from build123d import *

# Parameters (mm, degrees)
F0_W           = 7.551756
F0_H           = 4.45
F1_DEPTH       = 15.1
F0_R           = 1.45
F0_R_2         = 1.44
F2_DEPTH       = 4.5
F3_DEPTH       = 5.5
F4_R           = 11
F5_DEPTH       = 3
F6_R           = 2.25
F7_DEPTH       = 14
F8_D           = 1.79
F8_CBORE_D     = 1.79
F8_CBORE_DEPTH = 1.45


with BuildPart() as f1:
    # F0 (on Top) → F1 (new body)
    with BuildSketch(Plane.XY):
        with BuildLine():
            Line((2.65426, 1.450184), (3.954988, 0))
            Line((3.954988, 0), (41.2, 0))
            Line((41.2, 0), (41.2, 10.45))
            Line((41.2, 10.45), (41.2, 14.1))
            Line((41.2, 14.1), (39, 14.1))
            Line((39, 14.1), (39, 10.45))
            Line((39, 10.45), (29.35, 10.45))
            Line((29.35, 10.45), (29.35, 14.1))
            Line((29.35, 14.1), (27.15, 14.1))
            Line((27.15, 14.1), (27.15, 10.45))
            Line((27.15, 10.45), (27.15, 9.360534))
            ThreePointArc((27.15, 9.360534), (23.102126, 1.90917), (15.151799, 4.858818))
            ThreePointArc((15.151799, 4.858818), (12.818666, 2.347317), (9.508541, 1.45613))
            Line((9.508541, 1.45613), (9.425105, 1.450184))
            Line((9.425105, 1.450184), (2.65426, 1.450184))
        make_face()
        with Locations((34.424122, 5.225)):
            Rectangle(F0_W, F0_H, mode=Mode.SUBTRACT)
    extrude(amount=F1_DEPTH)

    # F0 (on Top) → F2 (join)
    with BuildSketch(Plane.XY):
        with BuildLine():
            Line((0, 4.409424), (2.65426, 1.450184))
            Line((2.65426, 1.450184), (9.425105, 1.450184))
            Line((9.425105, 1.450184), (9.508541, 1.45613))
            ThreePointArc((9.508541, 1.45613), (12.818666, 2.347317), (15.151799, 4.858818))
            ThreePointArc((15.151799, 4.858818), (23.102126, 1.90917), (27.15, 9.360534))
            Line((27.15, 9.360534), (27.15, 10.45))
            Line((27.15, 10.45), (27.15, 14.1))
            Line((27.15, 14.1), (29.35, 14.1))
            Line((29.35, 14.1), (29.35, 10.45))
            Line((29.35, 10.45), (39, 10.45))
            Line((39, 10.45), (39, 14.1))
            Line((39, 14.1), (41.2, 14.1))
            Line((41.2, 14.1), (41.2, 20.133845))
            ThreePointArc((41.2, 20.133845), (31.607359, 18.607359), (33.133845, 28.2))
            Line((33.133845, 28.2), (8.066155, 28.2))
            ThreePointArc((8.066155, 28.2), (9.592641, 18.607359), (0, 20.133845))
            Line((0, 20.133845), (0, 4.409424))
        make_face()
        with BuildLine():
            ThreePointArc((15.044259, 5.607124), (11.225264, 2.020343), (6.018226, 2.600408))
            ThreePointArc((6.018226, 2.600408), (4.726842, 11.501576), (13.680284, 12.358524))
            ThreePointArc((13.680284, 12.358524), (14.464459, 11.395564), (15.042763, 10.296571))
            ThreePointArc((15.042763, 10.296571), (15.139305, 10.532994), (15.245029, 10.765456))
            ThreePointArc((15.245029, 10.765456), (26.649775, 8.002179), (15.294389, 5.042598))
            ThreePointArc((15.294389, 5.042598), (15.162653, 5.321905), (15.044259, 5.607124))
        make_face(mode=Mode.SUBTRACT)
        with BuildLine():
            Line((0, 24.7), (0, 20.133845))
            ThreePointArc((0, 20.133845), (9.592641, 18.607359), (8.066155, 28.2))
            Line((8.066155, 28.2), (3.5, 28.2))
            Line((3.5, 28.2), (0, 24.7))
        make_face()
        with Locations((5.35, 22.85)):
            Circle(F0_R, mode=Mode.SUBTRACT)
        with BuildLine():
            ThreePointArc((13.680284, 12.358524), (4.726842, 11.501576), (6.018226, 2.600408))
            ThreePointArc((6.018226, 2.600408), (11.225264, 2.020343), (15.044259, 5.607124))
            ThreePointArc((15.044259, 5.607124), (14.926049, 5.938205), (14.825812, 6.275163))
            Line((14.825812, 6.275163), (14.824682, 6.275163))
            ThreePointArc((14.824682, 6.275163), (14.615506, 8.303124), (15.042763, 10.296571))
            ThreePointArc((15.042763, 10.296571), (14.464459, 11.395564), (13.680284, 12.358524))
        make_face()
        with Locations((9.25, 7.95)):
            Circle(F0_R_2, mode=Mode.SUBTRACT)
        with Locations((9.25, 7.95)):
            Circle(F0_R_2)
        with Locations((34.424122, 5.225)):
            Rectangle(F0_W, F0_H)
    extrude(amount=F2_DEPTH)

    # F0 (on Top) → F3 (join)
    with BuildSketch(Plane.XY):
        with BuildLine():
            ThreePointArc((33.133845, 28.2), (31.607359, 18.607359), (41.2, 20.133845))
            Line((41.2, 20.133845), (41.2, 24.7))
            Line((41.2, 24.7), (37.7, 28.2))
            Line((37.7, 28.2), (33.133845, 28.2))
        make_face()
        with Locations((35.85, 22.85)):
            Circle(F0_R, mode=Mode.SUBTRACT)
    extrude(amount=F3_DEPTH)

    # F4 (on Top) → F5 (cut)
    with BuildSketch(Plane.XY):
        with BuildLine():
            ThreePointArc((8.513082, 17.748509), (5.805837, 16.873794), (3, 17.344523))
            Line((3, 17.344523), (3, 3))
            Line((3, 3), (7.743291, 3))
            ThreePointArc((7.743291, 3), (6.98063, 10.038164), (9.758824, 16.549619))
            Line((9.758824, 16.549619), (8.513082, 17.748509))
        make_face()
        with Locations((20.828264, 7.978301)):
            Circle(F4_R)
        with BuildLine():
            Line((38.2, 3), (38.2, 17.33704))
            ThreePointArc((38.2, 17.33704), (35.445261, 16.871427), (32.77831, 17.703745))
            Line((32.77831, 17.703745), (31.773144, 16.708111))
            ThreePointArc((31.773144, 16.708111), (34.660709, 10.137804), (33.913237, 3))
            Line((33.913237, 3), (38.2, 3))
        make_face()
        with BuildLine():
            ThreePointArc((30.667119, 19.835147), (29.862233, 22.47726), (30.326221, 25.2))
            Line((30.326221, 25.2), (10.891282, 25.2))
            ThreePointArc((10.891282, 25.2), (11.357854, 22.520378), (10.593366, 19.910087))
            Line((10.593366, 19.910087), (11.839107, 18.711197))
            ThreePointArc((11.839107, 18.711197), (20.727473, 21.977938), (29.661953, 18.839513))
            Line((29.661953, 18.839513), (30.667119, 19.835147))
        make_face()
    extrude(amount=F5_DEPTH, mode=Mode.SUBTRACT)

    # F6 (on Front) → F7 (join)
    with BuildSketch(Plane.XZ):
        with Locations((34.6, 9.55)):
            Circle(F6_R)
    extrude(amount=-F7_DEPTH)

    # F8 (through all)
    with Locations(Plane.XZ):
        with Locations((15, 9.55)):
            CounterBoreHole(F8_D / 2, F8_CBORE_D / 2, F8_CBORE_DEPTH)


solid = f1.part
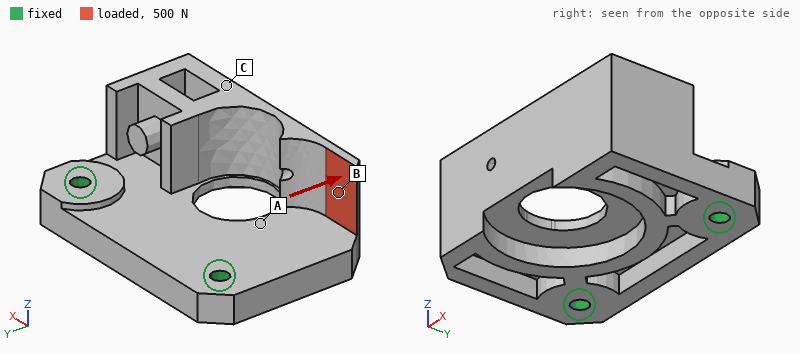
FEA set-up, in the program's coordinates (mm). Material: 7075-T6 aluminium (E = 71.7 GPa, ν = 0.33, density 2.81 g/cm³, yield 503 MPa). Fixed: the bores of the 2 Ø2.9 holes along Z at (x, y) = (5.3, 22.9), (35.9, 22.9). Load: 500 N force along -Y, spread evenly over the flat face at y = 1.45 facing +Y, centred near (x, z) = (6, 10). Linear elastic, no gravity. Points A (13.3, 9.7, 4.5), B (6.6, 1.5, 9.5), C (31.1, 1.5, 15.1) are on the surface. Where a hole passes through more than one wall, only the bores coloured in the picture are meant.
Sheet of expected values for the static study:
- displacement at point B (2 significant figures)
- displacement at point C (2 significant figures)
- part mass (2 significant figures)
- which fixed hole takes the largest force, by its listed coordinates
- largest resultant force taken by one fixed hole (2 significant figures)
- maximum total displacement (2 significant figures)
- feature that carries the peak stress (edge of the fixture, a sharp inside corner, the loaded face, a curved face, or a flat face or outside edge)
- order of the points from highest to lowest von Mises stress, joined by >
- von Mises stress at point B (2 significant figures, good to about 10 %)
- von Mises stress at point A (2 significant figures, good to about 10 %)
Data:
0.18 mm
0.078 mm
15 g
(5.3, 22.9)
470 N
0.44 mm
a flat face or outside edge
B > A > C
190 MPa
63 MPa
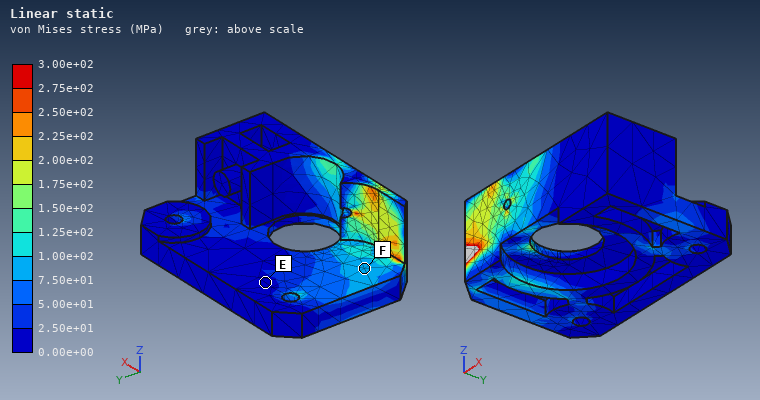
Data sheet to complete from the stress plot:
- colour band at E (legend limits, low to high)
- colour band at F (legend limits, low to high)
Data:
0.00e+00 to 2.50e+01 MPa
7.50e+01 to 1.00e+02 MPa
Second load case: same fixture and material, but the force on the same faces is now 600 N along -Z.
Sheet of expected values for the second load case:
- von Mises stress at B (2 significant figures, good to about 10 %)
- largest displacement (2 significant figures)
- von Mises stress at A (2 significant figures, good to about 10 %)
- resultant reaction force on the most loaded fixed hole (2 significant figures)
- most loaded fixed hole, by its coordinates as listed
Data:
74 MPa
0.34 mm
52 MPa
520 N
(5.3, 22.9)
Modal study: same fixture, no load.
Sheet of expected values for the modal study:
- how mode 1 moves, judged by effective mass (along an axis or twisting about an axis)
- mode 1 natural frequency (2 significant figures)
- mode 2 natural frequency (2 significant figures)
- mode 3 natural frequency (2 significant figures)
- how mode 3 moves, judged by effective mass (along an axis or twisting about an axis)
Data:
along Z
3500 Hz
6500 Hz
12 kHz
along X
